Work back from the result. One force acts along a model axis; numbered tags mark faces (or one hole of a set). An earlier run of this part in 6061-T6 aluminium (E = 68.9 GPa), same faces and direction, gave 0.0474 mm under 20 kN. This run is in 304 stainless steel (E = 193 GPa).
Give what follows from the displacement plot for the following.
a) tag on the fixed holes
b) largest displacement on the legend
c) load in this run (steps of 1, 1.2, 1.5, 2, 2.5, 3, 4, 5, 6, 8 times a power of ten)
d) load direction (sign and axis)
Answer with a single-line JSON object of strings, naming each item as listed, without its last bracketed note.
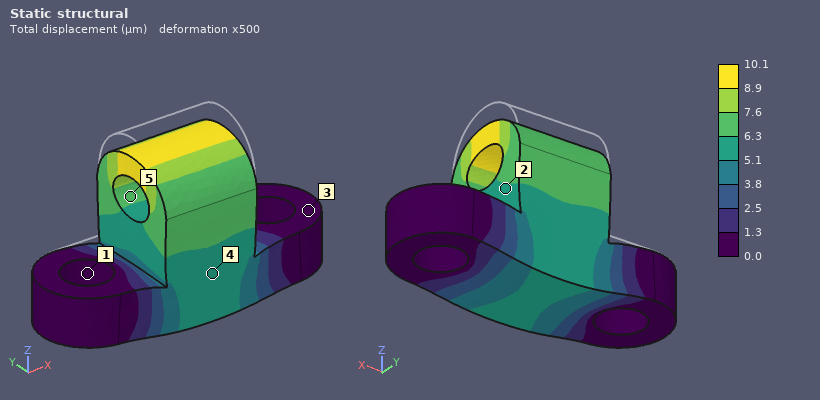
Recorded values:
{"tag on the fixed holes": "1", "largest displacement on the legend": "10.1 µm", "load in this run": "12 kN", "load direction": "-Z"}
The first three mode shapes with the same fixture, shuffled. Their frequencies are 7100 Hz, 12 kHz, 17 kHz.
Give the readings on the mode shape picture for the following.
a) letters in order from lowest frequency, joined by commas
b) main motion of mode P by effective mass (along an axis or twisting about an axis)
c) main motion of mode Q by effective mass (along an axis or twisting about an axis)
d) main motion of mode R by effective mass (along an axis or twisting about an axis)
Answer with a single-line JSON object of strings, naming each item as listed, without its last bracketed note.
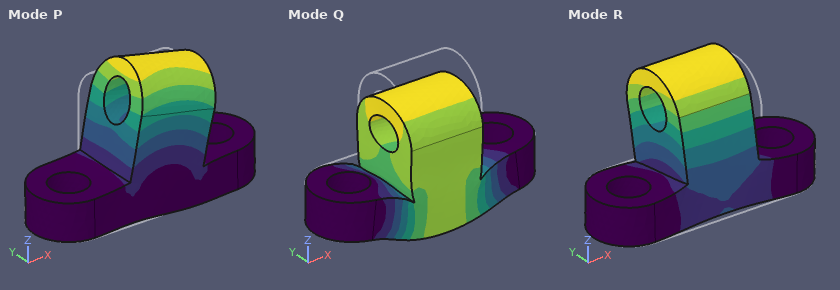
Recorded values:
{"letters in order from lowest frequency, joined by commas": "R, P, Q", "main motion of mode P by effective mass": "along X", "main motion of mode Q by effective mass": "along Z", "main motion of mode R by effective mass": "along Y"}
